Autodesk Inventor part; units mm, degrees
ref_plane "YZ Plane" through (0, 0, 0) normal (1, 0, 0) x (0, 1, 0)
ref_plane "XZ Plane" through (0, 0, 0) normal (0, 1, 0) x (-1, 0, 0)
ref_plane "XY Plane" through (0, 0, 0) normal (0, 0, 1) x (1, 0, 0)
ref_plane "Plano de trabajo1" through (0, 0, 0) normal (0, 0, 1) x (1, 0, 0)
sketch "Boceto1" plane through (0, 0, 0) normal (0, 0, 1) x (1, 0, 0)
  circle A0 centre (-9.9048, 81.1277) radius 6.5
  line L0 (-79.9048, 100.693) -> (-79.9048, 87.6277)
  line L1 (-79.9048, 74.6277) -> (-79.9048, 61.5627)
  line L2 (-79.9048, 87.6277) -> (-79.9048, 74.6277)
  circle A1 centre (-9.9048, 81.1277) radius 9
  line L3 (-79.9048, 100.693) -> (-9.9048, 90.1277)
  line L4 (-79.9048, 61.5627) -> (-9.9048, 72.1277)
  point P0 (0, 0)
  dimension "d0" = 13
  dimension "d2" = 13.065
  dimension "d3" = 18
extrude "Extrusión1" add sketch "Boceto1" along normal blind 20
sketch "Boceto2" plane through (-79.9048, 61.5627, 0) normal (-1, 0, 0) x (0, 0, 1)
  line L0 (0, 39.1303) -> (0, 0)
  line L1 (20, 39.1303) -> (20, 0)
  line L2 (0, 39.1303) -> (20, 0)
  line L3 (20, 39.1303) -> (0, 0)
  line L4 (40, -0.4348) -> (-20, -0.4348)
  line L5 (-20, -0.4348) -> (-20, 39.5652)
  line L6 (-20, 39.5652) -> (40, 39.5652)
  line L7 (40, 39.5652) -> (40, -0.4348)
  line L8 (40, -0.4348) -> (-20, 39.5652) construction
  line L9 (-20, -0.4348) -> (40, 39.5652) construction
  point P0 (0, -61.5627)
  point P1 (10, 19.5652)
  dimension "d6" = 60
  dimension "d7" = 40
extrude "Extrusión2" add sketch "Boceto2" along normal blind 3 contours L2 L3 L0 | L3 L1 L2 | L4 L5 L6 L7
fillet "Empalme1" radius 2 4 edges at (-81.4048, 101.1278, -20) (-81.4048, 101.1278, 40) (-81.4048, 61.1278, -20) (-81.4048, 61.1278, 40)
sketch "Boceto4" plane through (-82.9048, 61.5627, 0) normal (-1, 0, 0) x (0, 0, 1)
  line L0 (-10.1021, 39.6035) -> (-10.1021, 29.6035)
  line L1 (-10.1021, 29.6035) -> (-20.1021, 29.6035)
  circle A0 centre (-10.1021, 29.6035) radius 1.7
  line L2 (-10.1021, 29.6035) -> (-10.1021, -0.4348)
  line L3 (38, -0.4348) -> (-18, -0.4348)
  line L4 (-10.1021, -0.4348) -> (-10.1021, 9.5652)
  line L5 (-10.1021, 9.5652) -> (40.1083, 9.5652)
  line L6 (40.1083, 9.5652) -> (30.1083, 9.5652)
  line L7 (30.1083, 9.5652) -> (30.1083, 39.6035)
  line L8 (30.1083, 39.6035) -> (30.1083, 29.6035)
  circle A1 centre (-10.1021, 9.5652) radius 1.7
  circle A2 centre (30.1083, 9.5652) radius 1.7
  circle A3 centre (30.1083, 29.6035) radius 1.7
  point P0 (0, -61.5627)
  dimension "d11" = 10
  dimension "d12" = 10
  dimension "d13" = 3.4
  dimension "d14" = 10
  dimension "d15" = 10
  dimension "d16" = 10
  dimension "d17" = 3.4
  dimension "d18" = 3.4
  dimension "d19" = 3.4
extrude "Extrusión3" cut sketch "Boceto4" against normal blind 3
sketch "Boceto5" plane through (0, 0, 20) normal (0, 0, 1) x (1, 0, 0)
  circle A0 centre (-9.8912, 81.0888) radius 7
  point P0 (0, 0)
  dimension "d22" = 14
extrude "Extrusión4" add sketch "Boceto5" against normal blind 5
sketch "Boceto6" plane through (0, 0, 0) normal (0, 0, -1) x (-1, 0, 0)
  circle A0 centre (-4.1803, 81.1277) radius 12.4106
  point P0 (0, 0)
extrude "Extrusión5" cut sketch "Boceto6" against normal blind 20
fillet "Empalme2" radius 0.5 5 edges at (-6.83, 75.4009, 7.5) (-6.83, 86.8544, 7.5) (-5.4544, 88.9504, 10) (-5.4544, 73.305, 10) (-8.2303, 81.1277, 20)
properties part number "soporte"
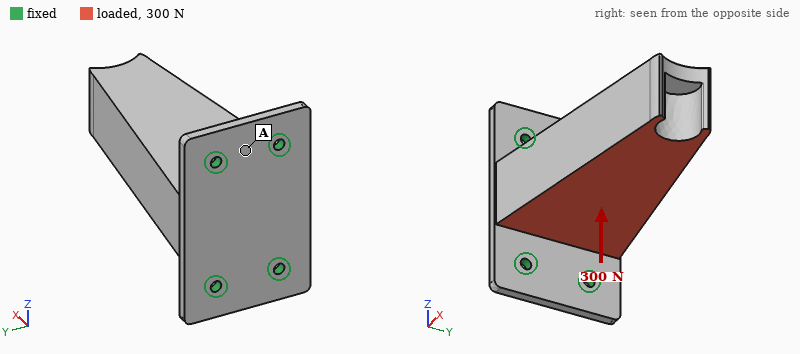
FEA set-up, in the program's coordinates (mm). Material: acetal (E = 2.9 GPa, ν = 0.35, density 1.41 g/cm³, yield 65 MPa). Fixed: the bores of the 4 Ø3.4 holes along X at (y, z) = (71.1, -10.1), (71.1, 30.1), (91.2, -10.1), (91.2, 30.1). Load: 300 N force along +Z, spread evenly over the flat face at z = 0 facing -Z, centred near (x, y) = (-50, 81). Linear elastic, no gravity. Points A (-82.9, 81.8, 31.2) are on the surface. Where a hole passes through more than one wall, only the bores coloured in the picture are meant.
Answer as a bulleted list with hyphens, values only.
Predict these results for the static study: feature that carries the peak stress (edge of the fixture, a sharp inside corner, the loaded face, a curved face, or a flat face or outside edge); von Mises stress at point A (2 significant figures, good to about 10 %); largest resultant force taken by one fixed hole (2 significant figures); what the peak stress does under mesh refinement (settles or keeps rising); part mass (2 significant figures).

- edge of the fixture
- 4.6 MPa
- 170 N
- keeps rising
- 66 g
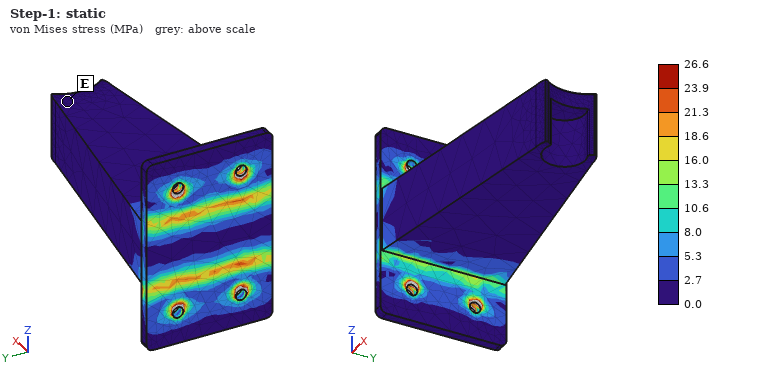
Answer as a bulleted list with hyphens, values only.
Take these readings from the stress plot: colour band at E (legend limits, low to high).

- 0.0 to 2.7 MPa
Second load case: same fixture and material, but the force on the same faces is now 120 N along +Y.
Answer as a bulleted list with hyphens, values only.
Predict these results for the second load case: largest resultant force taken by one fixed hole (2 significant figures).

- 96 N
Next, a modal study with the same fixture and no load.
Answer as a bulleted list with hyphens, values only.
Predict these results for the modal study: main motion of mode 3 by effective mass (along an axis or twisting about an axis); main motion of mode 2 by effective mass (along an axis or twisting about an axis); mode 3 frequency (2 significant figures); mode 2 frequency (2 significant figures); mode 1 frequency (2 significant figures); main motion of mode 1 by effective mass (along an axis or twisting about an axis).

- along X
- along Z
- 1100 Hz
- 440 Hz
- 340 Hz
- along Y
